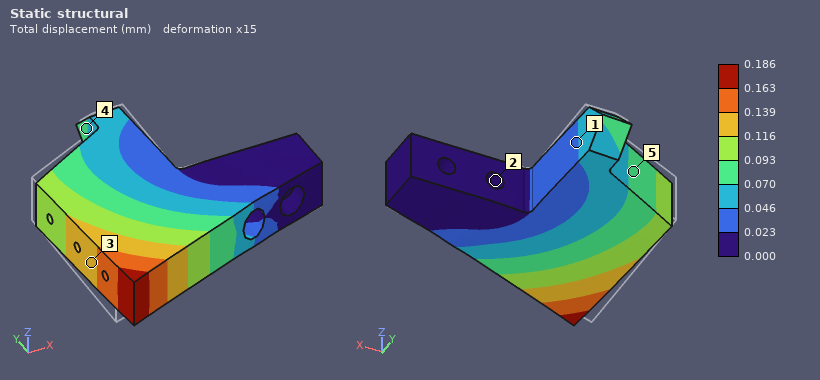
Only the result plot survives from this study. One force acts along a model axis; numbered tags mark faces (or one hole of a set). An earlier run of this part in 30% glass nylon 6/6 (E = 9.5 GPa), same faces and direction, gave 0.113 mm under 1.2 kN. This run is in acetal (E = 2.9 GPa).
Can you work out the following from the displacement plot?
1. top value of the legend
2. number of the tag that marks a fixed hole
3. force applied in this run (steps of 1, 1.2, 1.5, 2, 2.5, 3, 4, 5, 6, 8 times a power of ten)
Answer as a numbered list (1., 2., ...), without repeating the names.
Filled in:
1. 0.186 mm
2. 2
3. 600 N
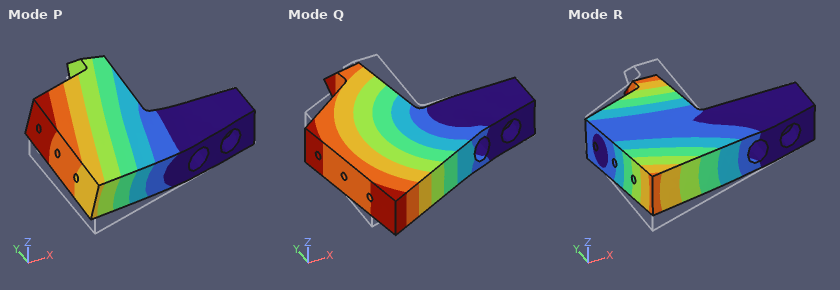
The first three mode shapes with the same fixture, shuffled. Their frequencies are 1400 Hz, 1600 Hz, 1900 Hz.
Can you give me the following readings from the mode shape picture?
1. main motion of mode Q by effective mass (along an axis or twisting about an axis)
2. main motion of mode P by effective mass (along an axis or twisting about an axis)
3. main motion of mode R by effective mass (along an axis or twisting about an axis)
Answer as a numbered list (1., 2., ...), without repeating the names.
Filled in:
1. along Y
2. along Z
3. twisting about X
